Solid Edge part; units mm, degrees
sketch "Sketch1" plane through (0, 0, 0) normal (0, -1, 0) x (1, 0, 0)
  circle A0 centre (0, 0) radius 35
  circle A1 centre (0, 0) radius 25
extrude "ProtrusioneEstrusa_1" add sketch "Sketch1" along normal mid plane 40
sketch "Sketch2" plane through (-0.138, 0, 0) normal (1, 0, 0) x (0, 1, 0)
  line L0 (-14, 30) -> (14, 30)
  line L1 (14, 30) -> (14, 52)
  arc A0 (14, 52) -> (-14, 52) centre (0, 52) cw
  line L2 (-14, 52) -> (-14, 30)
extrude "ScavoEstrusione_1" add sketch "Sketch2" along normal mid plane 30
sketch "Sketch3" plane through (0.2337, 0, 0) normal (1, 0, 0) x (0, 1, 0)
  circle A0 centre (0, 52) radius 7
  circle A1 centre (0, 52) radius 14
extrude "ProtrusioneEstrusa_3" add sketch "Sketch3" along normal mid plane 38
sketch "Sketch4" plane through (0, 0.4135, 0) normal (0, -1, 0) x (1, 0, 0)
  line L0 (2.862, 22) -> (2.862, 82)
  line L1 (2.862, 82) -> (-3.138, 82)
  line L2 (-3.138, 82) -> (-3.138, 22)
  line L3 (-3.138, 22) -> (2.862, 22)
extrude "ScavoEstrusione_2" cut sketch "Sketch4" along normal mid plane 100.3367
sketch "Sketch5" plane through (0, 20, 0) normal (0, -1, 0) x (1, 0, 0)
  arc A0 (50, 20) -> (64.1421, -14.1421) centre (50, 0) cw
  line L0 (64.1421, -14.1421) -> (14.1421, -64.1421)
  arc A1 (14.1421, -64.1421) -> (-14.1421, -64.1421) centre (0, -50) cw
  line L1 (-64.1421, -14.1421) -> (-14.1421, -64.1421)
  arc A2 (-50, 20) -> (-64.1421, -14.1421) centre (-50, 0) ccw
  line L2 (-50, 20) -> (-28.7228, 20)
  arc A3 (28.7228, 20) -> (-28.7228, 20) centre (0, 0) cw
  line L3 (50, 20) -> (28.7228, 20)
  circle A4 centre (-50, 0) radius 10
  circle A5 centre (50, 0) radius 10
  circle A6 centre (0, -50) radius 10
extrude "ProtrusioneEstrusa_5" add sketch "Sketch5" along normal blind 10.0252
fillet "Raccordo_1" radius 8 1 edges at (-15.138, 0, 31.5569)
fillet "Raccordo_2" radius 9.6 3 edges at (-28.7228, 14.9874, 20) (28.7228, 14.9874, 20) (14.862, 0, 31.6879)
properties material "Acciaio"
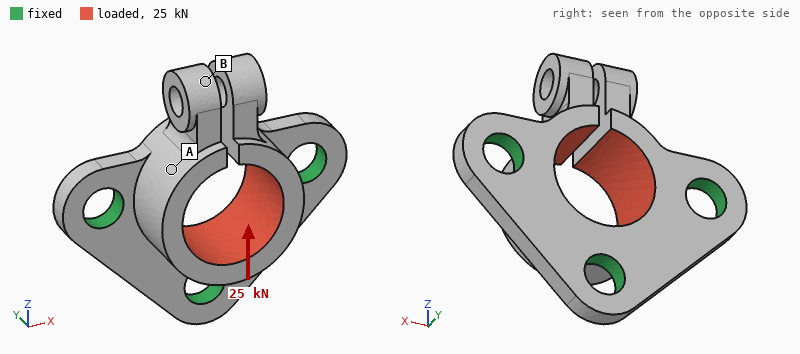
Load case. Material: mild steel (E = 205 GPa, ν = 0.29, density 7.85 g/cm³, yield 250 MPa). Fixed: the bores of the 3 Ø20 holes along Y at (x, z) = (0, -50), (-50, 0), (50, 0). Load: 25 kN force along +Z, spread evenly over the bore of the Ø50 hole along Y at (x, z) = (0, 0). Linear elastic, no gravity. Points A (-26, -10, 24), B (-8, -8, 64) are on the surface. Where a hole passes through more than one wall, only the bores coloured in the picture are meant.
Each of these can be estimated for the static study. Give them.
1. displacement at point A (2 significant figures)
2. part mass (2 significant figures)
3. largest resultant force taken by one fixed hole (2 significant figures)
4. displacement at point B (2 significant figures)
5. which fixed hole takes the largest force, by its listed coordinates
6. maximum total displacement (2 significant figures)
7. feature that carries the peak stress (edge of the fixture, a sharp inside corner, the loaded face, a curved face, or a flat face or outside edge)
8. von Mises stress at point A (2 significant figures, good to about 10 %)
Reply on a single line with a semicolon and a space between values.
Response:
0.031 mm; 1.1 kg; 13 kN; 0.10 mm; (0, -50); 0.11 mm; a curved face; 26 MPa
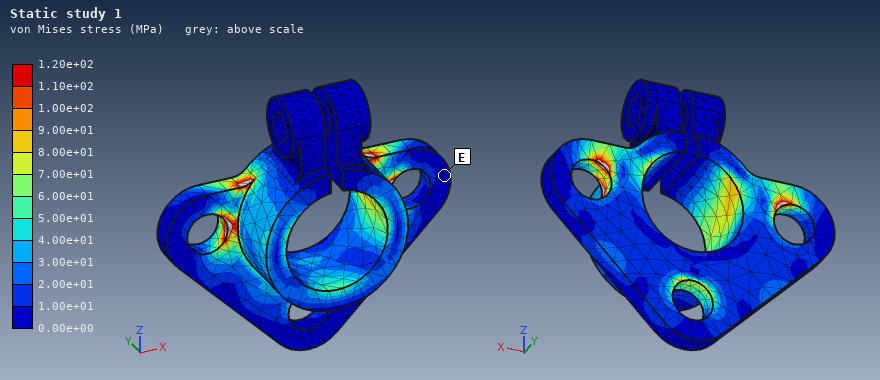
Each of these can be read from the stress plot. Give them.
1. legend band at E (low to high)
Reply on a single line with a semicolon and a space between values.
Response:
0.00e+00 to 1.00e+01 MPa
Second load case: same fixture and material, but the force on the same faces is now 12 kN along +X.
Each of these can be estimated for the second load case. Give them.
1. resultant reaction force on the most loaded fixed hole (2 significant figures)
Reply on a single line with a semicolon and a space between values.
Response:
4.9 kN
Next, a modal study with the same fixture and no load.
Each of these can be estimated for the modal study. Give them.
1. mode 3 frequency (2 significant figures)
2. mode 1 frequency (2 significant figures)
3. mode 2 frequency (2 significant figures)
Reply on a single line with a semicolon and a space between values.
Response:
2500 Hz; 1900 Hz; 1900 Hz
